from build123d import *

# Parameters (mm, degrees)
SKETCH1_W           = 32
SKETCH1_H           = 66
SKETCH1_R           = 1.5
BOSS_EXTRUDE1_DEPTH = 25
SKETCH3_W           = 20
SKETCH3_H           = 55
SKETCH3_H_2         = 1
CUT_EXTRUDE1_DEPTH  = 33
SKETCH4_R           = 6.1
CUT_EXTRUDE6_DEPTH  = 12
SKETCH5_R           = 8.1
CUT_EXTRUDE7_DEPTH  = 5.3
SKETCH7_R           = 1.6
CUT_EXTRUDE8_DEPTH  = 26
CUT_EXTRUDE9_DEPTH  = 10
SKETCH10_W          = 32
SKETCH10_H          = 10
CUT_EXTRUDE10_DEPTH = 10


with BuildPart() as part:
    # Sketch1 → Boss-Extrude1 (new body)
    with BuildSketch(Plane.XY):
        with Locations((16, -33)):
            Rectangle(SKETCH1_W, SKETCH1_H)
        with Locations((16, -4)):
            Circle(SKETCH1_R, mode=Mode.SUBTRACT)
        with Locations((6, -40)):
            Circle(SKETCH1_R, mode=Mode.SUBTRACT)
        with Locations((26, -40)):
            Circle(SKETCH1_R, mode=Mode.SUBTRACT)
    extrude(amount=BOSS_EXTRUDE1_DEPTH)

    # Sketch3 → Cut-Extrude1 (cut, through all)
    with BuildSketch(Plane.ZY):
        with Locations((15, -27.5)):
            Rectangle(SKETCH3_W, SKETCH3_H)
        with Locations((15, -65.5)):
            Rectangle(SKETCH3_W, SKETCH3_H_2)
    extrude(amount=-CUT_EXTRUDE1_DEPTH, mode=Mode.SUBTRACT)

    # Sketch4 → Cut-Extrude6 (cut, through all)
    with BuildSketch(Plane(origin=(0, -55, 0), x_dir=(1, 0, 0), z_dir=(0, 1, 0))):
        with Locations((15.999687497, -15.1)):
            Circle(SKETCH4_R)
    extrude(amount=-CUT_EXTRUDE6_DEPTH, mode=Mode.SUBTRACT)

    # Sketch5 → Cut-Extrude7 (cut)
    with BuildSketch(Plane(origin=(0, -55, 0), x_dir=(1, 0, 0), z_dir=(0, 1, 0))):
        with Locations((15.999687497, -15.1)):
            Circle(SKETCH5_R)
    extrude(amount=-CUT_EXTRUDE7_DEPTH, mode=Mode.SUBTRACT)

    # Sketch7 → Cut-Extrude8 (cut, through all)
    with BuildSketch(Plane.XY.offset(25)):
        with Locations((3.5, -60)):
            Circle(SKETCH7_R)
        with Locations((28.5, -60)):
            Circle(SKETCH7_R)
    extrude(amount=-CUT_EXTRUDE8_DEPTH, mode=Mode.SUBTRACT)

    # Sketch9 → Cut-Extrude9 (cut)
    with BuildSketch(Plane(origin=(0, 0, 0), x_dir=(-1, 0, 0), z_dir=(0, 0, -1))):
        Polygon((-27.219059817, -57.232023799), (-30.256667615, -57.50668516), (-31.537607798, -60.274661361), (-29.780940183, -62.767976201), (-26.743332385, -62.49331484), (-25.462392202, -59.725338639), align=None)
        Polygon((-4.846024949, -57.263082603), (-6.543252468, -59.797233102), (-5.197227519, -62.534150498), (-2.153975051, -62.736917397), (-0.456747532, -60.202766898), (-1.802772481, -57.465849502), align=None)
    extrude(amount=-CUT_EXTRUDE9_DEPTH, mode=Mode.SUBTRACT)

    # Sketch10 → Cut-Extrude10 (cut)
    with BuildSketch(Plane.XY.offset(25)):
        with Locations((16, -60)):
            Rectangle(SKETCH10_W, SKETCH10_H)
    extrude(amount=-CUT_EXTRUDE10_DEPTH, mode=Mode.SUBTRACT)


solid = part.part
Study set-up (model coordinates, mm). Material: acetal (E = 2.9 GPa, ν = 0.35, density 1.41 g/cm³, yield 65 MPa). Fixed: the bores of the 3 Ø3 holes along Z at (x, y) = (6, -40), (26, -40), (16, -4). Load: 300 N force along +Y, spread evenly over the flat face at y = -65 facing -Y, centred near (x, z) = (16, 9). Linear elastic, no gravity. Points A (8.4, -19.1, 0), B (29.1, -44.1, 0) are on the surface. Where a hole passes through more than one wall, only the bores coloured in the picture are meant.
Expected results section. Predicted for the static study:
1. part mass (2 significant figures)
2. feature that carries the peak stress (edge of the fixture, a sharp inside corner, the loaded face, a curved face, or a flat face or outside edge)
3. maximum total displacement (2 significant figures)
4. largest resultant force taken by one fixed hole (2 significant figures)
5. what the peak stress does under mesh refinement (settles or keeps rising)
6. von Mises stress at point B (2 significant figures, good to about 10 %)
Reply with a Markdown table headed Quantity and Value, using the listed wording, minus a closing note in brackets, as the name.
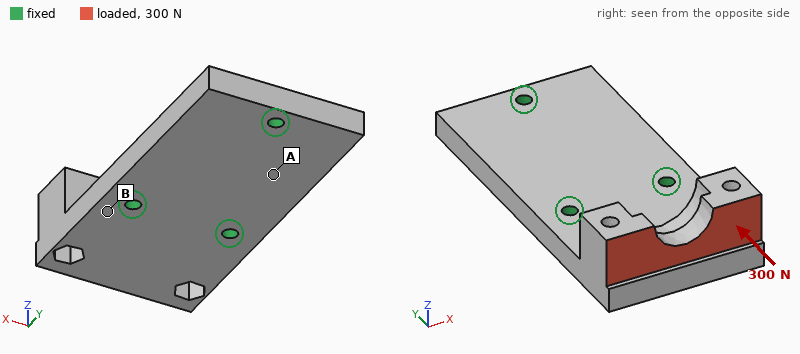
| Quantity | Value |
|---|---|
| part mass | 17 g |
| feature that carries the peak stress | edge of the fixture |
| maximum total displacement | 0.81 mm |
| largest resultant force taken by one fixed hole | 140 N |
| what the peak stress does under mesh refinement | keeps rising |
| von Mises stress at point B | 13 MPa |
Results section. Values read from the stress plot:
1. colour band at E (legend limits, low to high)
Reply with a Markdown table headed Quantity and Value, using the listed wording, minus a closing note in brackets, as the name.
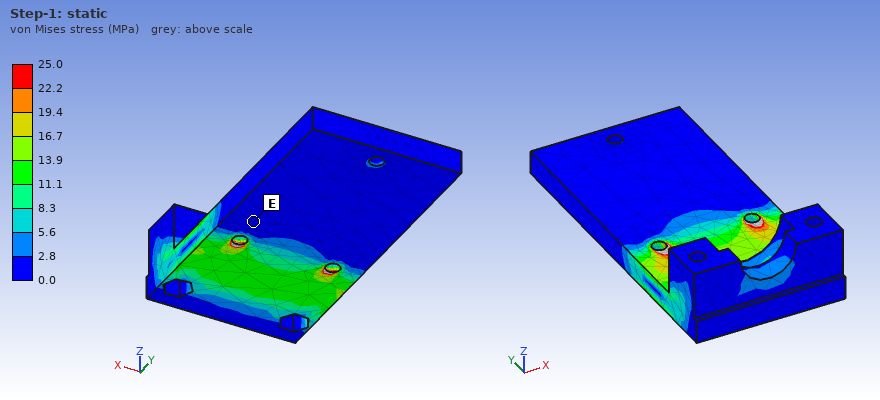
| Quantity | Value |
|---|---|
| colour band at E | 0.0 to 2.8 MPa |
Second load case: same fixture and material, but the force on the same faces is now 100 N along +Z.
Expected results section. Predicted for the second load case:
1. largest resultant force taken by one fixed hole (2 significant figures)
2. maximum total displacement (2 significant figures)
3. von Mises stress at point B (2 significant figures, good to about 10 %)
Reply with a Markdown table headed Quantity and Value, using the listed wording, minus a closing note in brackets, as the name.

| Quantity | Value |
|---|---|
| largest resultant force taken by one fixed hole | 56 N |
| maximum total displacement | 0.69 mm |
| von Mises stress at point B | 15 MPa |
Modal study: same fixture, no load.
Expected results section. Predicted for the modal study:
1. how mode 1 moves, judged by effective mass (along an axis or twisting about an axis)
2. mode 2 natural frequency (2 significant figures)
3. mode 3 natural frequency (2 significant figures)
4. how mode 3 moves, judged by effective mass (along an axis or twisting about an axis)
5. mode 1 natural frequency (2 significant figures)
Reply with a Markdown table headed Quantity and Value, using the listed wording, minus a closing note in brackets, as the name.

| Quantity | Value |
|---|---|
| how mode 1 moves, judged by effective mass | along Z |
| mode 2 natural frequency | 2400 Hz |
| mode 3 natural frequency | 3500 Hz |
| how mode 3 moves, judged by effective mass | twisting about Y |
| mode 1 natural frequency | 1100 Hz |
